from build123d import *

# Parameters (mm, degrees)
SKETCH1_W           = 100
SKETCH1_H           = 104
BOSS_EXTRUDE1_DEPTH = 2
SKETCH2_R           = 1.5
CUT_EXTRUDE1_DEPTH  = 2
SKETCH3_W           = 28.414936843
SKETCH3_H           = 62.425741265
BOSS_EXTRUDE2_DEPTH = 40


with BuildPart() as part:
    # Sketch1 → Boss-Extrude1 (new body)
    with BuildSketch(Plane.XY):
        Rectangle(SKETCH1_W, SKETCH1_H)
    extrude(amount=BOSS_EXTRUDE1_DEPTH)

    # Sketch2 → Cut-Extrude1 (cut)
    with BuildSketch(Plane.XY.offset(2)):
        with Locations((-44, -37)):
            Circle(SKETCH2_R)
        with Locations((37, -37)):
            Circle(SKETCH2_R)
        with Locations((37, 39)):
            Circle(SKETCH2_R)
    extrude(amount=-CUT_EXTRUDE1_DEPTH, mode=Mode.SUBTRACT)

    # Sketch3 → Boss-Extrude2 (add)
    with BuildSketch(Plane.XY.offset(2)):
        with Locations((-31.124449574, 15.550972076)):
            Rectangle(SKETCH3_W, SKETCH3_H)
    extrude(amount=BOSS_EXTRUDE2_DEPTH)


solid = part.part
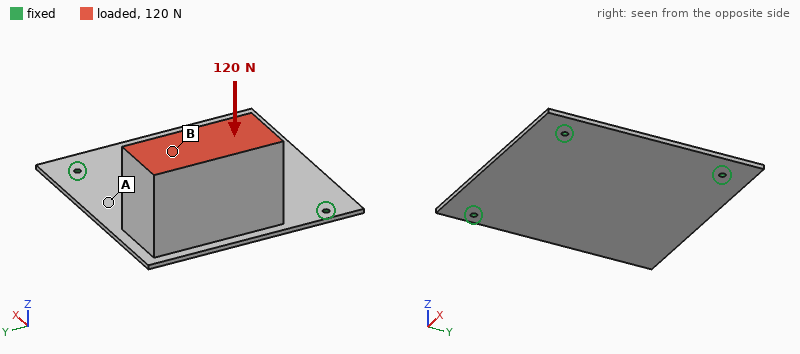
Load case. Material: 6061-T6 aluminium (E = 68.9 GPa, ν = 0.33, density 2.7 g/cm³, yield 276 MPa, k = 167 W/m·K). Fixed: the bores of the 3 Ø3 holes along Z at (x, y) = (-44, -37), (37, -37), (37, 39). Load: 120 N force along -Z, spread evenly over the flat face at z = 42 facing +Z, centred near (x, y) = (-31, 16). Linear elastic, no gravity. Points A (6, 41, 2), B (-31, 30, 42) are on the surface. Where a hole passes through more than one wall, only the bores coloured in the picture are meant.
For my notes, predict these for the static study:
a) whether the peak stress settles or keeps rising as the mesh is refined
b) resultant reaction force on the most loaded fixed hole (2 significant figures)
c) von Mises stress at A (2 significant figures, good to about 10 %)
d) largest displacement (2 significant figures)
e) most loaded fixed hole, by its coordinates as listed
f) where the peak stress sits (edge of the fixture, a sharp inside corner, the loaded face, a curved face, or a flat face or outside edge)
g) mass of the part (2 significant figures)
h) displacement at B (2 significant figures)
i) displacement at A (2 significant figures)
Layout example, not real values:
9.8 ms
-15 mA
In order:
keeps rising
84 N
23 MPa
0.96 mm
(-44, -37)
edge of the fixture
250 g
0.76 mm
0.35 mm
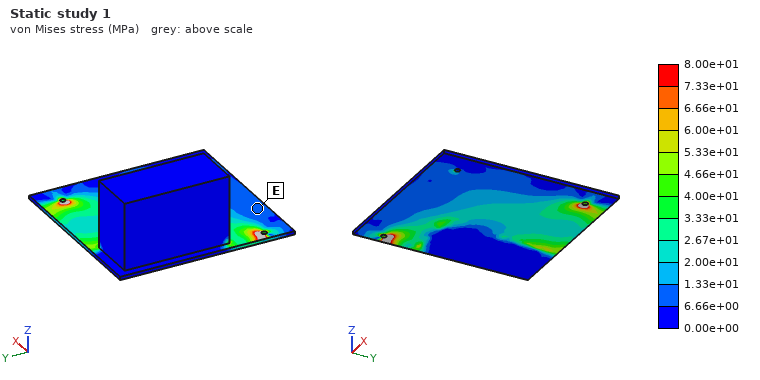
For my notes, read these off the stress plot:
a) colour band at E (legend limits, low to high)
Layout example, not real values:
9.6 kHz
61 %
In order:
6.66e+00 to 1.33e+01 MPa
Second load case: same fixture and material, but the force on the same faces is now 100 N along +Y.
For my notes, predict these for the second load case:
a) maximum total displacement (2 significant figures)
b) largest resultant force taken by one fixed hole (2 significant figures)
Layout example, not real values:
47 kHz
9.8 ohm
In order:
0.80 mm
62 N
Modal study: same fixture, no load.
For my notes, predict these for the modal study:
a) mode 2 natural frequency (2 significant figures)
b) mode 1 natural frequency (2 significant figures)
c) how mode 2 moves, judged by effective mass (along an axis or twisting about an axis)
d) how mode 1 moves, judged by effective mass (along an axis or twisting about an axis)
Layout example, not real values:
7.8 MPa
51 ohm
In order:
370 Hz
140 Hz
along X
along Z
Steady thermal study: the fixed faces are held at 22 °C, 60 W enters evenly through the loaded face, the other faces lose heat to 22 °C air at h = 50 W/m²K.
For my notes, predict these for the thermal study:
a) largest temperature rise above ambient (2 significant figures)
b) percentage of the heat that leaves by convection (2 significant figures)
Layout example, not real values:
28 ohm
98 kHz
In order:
50 K
60 %
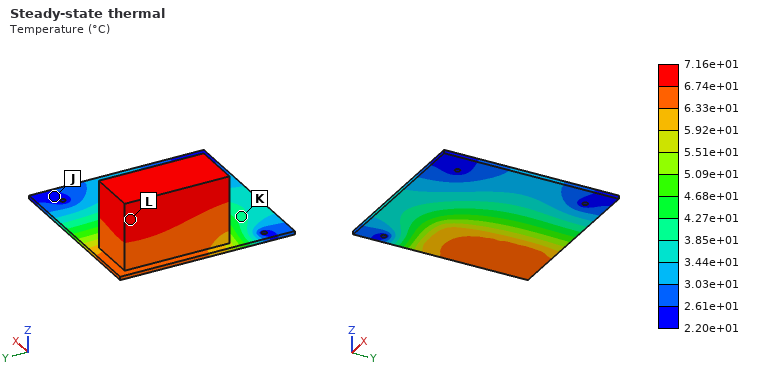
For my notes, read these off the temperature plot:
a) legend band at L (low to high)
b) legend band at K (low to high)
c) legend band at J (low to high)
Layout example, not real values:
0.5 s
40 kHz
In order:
6.74e+01 to 7.16e+01 °C
3.85e+01 to 4.27e+01 °C
2.20e+01 to 2.61e+01 °C
